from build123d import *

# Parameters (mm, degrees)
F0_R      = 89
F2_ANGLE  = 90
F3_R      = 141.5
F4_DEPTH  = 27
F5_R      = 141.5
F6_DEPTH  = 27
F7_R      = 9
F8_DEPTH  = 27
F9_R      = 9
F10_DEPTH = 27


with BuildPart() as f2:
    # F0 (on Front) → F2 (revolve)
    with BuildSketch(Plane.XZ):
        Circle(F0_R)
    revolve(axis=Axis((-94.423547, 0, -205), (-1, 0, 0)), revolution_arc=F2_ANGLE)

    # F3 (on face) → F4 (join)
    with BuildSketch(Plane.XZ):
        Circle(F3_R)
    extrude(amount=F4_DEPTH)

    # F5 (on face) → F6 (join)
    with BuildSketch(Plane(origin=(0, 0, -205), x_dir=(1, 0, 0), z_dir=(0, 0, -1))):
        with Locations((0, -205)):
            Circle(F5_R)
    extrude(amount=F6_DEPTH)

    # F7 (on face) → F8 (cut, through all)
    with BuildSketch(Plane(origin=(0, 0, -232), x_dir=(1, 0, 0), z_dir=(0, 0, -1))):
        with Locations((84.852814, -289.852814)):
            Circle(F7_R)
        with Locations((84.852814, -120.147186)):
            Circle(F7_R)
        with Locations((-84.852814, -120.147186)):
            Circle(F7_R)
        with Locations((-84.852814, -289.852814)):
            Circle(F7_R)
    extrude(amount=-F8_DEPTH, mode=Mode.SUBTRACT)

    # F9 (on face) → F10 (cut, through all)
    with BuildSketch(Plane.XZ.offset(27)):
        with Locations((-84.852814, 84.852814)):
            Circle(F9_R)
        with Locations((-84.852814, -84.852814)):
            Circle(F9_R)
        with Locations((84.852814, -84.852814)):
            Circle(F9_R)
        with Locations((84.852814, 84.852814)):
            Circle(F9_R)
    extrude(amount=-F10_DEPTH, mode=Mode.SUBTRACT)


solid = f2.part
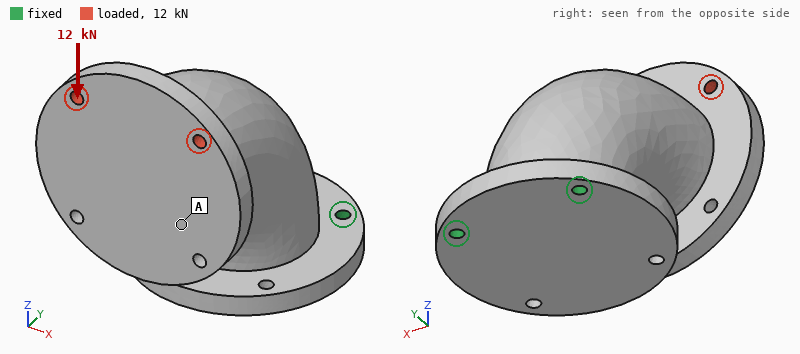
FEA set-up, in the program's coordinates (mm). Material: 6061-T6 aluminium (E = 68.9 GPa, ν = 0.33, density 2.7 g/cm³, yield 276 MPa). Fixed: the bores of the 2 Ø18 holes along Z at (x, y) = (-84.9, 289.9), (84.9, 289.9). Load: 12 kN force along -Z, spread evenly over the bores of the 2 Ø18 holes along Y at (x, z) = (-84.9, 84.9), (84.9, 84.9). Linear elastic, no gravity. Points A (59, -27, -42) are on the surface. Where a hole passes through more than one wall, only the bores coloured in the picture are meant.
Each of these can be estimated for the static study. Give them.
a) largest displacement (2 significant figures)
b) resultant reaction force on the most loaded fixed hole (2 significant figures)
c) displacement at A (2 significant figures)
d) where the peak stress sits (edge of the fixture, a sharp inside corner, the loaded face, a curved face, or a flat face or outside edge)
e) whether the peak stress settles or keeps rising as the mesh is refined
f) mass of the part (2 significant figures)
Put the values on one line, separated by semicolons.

2.6 mm; 6.0 kN; 2.0 mm; edge of the fixture; keeps rising; 31 kg
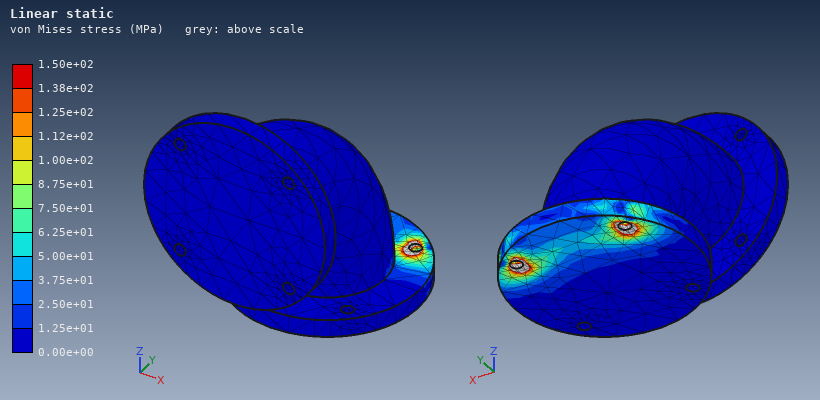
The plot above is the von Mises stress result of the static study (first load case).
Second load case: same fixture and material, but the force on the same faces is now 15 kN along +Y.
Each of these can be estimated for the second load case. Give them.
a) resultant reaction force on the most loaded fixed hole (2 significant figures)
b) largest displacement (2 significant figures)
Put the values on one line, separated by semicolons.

7.7 kN; 3.4 mm
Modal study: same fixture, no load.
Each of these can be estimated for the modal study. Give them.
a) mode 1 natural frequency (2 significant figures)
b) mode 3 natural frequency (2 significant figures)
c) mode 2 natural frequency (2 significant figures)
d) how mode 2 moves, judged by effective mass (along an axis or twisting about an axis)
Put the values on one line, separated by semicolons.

94 Hz; 1000 Hz; 350 Hz; along X
